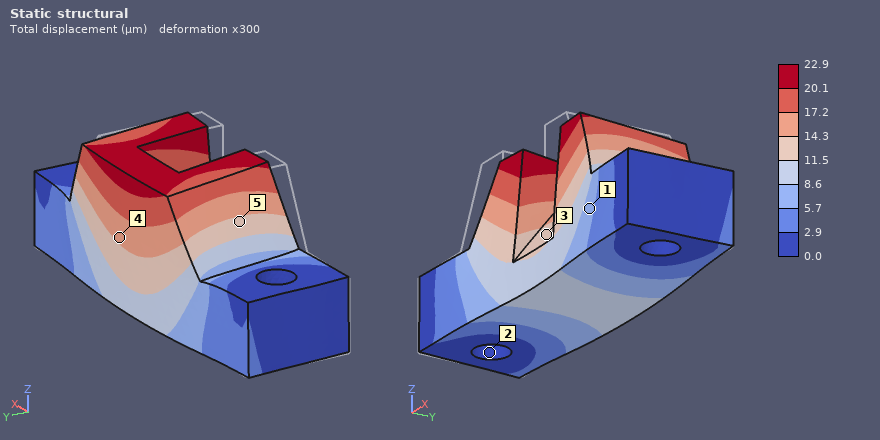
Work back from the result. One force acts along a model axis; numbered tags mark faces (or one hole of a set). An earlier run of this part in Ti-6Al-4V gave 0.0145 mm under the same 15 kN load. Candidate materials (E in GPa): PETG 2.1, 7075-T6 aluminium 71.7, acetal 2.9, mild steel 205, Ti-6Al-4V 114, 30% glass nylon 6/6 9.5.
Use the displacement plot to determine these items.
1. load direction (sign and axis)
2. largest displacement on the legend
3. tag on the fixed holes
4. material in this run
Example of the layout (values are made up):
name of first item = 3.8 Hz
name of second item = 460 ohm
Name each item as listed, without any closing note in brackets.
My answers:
load direction = +Y
largest displacement on the legend = 22.9 µm
tag on the fixed holes = 2
material in this run = 7075-T6 aluminium
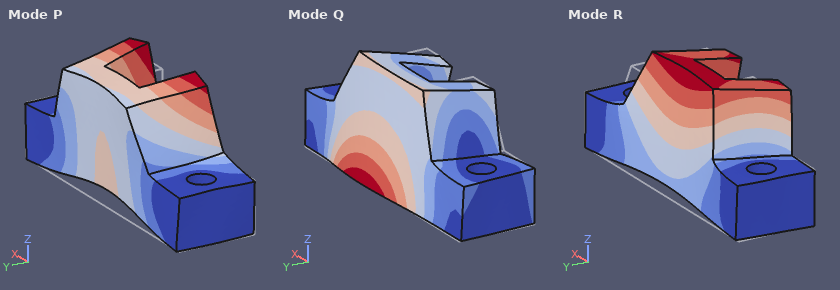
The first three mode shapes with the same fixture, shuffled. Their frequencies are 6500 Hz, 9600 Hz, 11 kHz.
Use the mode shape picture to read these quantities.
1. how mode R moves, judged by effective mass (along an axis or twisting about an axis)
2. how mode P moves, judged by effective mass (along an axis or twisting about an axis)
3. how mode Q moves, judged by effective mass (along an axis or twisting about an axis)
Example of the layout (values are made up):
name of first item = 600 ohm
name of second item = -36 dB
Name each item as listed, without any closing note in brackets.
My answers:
how mode R moves, judged by effective mass = along Y
how mode P moves, judged by effective mass = along Z
how mode Q moves, judged by effective mass = along Y
